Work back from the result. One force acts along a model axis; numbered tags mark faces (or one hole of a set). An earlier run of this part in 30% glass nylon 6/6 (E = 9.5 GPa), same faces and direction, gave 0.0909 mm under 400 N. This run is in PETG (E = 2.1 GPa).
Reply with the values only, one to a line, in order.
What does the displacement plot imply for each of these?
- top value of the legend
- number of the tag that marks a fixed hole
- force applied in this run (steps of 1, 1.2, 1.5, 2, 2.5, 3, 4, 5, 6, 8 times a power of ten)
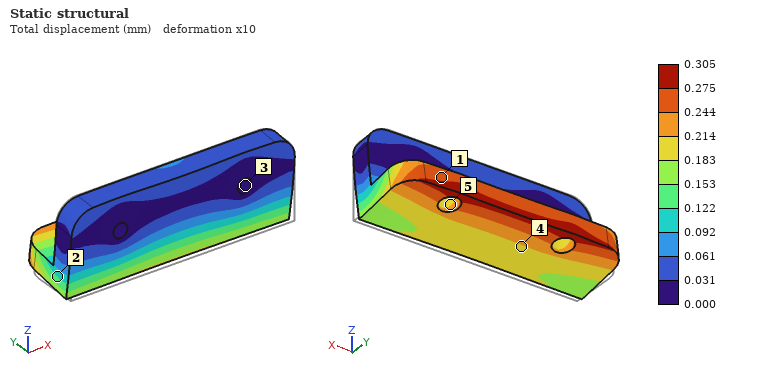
0.305 mm
3
300 N
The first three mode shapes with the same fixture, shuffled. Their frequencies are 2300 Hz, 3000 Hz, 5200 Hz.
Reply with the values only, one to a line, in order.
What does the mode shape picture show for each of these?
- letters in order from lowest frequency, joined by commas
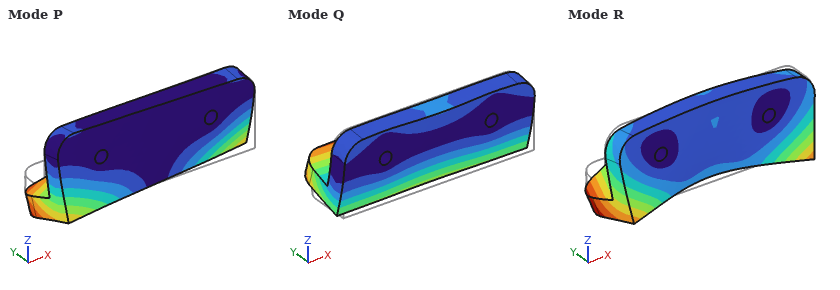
Q, P, R
